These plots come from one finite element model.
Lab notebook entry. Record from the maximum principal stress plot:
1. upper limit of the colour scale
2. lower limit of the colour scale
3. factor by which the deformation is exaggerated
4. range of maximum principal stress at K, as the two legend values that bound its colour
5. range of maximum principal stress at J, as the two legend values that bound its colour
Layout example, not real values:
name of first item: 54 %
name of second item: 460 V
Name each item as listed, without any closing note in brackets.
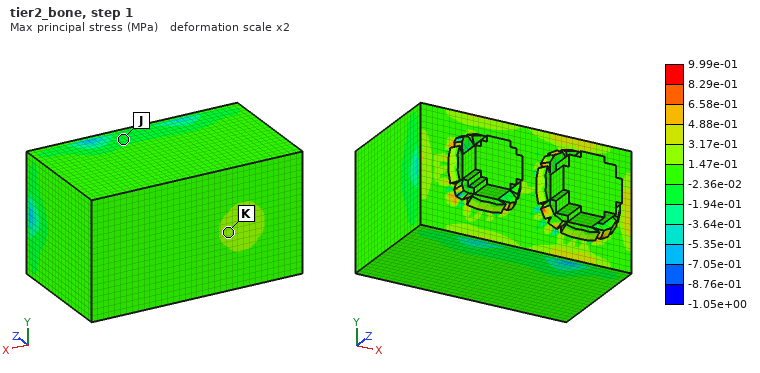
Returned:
upper limit of the colour scale: 9.99e-01 MPa
lower limit of the colour scale: -1.05e+00 MPa
factor by which the deformation is exaggerated: 2
range of maximum principal stress at K, as the two legend values that bound its colour: 1.47e-01 to 3.17e-01 MPa
range of maximum principal stress at J, as the two legend values that bound its colour: -1.94e-01 to -2.36e-02 MPa
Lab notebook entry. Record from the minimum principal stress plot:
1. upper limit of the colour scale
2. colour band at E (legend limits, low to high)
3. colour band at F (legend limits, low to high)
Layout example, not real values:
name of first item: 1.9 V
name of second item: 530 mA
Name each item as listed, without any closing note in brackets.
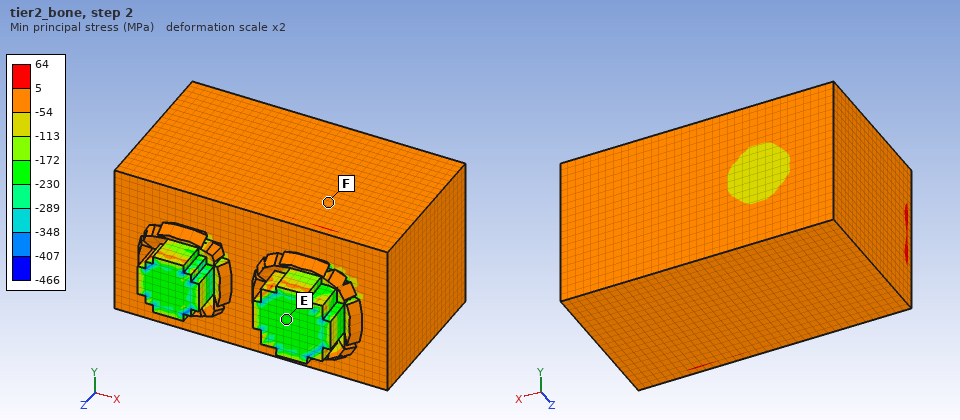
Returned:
upper limit of the colour scale: 64 MPa
colour band at E: -230 to -172 MPa
colour band at F: -54 to 5 MPa
